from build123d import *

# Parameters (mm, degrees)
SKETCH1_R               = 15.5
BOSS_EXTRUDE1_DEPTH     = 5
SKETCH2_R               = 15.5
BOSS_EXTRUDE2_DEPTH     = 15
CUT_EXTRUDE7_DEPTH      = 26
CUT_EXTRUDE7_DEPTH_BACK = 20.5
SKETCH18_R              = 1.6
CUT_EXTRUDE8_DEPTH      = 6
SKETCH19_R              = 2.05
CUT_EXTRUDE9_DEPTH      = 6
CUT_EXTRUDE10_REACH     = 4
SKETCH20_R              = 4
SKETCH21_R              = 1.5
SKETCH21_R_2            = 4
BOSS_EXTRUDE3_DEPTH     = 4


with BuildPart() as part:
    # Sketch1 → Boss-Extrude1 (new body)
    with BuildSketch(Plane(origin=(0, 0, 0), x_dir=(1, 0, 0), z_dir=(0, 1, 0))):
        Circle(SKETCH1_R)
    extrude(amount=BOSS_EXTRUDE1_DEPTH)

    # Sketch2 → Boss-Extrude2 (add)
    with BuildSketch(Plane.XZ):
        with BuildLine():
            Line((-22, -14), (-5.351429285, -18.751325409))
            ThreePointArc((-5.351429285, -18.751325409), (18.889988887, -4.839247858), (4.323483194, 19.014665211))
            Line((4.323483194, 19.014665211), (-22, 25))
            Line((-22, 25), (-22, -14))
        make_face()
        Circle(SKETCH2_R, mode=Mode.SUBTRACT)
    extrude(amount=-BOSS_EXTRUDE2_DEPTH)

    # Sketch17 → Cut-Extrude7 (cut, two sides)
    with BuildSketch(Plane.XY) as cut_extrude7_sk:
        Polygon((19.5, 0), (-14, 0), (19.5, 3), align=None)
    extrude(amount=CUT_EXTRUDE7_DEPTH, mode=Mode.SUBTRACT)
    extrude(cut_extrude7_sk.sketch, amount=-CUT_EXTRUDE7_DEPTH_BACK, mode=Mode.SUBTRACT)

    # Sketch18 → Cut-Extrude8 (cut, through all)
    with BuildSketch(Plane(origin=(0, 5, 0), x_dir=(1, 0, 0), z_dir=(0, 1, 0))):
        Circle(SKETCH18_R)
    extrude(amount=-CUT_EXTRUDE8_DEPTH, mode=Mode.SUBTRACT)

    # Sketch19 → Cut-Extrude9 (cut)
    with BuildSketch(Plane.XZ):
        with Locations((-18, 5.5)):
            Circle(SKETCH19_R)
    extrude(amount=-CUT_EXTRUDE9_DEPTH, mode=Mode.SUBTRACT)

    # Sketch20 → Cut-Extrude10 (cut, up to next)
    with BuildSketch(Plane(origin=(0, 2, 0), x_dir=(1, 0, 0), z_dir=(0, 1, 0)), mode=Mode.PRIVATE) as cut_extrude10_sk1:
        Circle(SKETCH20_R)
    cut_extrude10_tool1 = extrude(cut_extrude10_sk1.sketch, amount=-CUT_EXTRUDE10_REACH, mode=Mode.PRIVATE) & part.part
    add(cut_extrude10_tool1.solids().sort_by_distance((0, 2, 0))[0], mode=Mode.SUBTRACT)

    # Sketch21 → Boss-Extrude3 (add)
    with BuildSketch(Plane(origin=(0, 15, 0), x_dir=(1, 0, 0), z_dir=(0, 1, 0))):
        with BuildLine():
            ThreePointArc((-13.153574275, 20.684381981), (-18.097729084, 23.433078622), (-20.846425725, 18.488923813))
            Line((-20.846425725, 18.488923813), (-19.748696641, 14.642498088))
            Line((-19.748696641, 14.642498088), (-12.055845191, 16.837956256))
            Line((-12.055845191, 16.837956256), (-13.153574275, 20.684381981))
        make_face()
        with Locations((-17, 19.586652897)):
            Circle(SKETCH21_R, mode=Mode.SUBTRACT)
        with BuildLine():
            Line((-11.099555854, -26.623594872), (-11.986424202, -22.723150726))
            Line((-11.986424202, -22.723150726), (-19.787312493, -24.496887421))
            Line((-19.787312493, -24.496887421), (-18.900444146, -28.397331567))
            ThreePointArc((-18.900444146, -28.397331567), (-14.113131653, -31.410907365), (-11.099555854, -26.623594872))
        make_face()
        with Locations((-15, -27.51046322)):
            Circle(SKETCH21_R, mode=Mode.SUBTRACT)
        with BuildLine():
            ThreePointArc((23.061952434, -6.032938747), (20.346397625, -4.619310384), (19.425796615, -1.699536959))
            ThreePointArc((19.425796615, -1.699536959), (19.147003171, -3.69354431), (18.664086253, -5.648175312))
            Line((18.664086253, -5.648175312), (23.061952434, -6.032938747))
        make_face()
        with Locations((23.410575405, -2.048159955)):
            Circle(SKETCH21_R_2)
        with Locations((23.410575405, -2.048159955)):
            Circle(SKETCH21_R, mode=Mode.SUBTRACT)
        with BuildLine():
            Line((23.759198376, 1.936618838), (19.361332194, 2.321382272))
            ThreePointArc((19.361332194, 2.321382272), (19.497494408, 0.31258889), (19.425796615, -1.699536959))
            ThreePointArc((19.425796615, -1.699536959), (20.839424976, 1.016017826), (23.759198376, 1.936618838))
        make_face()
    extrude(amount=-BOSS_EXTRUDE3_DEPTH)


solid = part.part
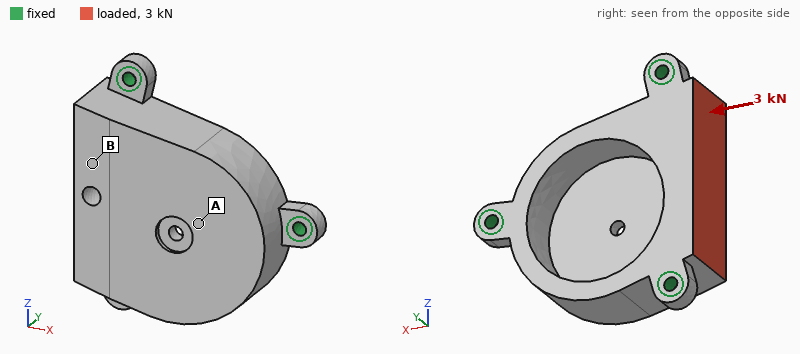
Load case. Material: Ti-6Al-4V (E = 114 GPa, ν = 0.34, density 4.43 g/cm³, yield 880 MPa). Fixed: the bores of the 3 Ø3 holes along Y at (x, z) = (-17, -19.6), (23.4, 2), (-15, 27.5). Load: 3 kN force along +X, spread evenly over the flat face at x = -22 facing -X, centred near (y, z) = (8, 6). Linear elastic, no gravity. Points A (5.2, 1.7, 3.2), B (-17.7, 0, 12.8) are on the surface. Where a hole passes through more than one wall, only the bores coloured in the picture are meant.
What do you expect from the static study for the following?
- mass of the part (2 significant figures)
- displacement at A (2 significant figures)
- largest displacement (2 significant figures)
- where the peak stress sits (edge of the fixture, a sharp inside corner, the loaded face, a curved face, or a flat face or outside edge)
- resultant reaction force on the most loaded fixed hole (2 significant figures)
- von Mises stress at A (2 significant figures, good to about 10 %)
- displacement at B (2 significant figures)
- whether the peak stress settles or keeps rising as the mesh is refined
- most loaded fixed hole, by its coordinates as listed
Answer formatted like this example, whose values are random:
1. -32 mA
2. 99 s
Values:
1. 59 g
2. 9.1 µm
3. 14 µm
4. edge of the fixture
5. 1.2 kN
6. 19 MPa
7. 11 µm
8. keeps rising
9. (-15, 27.5)
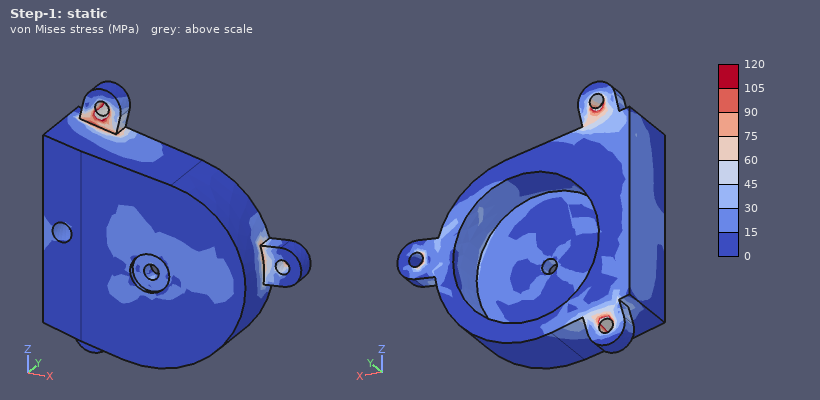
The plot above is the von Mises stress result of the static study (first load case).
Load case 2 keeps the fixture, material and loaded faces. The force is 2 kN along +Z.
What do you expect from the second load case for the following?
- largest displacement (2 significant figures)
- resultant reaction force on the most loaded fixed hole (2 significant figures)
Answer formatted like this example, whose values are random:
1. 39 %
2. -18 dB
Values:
1. 5.8 µm
2. 1.1 kN
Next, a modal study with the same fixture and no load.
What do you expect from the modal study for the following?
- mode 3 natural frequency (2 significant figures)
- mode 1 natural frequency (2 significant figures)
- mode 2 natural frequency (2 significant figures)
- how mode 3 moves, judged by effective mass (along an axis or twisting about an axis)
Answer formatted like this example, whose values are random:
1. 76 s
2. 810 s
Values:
1. 13 kHz
2. 12 kHz
3. 12 kHz
4. along X
